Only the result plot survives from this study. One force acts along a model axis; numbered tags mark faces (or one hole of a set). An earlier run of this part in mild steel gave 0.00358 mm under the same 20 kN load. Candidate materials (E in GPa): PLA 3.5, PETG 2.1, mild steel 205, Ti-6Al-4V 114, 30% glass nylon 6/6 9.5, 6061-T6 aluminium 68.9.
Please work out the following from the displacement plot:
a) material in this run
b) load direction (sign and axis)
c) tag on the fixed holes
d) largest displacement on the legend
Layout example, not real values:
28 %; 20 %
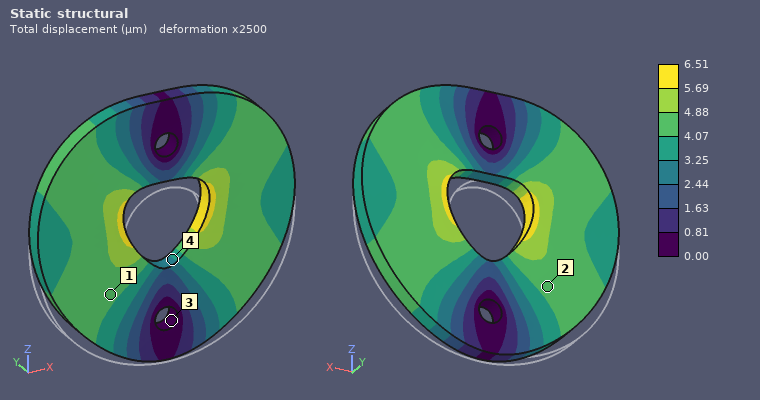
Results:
Ti-6Al-4V; +Z; 3; 6.51 µm
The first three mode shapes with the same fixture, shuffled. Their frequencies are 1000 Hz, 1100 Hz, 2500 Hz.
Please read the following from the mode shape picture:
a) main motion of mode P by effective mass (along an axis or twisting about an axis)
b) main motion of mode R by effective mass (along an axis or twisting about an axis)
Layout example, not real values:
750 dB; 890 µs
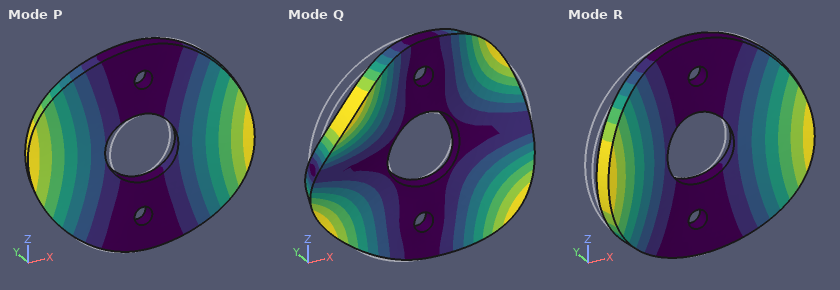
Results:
twisting about Z; along Y
